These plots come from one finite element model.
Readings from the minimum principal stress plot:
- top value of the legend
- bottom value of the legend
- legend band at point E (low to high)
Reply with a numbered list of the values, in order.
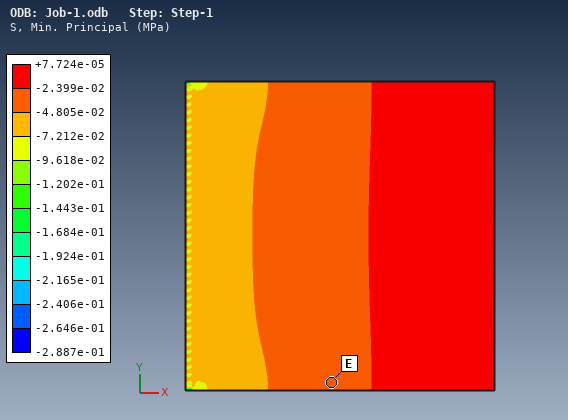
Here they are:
1. +7.724e-05 MPa
2. -2.887e-01 MPa
3. -4.805e-02 to -2.399e-02 MPa
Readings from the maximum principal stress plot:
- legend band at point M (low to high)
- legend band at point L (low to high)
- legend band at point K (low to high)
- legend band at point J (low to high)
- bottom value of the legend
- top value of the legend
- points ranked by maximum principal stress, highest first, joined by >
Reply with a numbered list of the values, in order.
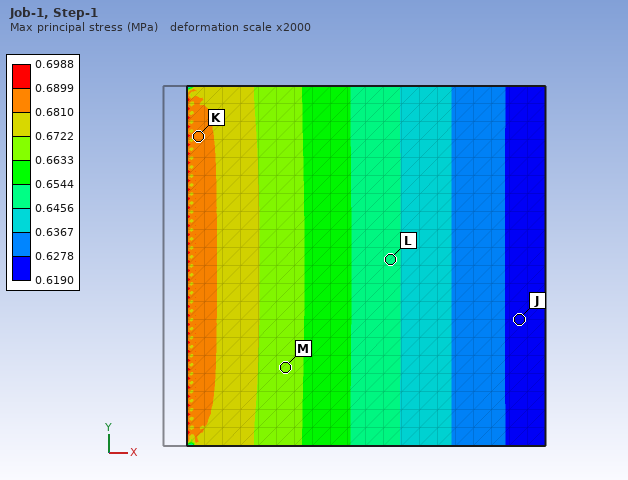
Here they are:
1. 0.6633 to 0.6722 MPa
2. 0.6456 to 0.6544 MPa
3. 0.6810 to 0.6899 MPa
4. 0.6190 to 0.6278 MPa
5. 0.6190 MPa
6. 0.6988 MPa
7. K > M > L > J
